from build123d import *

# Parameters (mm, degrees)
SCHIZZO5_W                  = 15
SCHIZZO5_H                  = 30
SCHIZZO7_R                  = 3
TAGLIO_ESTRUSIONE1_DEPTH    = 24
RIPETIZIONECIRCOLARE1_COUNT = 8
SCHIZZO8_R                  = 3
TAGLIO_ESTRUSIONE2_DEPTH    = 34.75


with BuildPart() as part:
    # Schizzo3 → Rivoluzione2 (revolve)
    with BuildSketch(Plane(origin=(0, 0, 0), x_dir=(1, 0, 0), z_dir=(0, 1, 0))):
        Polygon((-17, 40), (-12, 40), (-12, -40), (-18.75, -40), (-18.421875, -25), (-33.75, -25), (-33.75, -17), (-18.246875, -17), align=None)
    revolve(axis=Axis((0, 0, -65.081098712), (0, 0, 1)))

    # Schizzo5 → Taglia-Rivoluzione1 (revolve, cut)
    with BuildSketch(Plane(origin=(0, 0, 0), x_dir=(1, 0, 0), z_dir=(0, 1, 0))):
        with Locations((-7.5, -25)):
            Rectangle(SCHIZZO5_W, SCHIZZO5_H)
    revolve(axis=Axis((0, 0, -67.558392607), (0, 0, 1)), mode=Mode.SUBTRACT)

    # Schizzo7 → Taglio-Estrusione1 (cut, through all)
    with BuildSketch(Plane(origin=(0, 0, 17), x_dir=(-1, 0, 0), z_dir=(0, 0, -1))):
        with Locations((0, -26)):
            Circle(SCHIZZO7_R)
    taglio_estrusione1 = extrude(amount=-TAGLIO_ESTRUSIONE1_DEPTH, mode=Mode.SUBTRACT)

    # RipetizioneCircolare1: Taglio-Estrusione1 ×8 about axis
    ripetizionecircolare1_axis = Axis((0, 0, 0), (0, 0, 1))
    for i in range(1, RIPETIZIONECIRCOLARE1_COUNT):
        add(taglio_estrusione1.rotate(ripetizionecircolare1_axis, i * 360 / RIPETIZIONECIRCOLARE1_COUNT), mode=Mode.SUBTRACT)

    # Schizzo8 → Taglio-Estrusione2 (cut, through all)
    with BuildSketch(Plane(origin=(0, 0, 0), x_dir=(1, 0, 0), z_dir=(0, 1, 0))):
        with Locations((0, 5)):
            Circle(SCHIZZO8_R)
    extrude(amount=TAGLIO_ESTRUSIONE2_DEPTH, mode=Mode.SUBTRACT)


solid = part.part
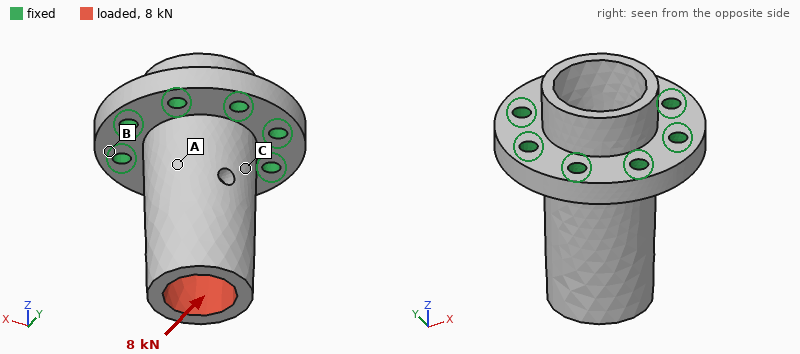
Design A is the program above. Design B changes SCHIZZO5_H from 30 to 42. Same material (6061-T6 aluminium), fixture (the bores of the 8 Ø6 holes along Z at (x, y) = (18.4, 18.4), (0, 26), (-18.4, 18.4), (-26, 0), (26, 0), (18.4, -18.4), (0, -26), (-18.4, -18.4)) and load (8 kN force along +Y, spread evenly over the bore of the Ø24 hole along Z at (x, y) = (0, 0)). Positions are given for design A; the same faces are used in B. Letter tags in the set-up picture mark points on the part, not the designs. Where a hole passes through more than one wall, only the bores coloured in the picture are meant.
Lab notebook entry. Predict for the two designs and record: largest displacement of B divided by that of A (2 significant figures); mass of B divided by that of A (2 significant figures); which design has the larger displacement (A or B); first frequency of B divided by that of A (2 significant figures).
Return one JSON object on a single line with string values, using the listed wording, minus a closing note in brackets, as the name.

{"largest displacement of B divided by that of A": "1.2", "mass of B divided by that of A": "0.97", "which design has the larger displacement": "B", "first frequency of B divided by that of A": "0.95"}
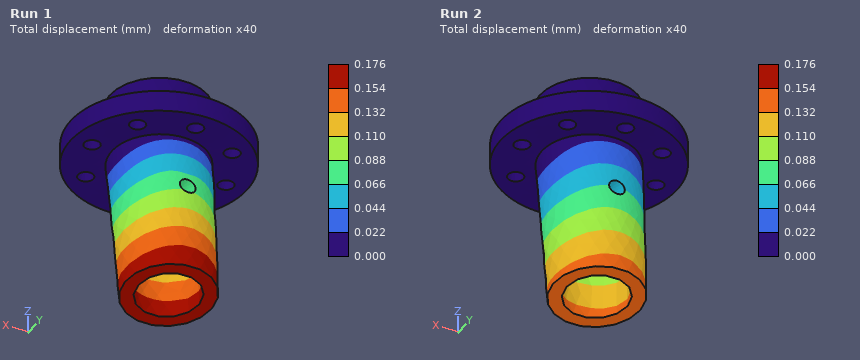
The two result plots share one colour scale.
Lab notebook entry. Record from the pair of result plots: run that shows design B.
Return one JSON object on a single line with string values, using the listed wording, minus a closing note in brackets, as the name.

{"run that shows design B": "Run 1"}
